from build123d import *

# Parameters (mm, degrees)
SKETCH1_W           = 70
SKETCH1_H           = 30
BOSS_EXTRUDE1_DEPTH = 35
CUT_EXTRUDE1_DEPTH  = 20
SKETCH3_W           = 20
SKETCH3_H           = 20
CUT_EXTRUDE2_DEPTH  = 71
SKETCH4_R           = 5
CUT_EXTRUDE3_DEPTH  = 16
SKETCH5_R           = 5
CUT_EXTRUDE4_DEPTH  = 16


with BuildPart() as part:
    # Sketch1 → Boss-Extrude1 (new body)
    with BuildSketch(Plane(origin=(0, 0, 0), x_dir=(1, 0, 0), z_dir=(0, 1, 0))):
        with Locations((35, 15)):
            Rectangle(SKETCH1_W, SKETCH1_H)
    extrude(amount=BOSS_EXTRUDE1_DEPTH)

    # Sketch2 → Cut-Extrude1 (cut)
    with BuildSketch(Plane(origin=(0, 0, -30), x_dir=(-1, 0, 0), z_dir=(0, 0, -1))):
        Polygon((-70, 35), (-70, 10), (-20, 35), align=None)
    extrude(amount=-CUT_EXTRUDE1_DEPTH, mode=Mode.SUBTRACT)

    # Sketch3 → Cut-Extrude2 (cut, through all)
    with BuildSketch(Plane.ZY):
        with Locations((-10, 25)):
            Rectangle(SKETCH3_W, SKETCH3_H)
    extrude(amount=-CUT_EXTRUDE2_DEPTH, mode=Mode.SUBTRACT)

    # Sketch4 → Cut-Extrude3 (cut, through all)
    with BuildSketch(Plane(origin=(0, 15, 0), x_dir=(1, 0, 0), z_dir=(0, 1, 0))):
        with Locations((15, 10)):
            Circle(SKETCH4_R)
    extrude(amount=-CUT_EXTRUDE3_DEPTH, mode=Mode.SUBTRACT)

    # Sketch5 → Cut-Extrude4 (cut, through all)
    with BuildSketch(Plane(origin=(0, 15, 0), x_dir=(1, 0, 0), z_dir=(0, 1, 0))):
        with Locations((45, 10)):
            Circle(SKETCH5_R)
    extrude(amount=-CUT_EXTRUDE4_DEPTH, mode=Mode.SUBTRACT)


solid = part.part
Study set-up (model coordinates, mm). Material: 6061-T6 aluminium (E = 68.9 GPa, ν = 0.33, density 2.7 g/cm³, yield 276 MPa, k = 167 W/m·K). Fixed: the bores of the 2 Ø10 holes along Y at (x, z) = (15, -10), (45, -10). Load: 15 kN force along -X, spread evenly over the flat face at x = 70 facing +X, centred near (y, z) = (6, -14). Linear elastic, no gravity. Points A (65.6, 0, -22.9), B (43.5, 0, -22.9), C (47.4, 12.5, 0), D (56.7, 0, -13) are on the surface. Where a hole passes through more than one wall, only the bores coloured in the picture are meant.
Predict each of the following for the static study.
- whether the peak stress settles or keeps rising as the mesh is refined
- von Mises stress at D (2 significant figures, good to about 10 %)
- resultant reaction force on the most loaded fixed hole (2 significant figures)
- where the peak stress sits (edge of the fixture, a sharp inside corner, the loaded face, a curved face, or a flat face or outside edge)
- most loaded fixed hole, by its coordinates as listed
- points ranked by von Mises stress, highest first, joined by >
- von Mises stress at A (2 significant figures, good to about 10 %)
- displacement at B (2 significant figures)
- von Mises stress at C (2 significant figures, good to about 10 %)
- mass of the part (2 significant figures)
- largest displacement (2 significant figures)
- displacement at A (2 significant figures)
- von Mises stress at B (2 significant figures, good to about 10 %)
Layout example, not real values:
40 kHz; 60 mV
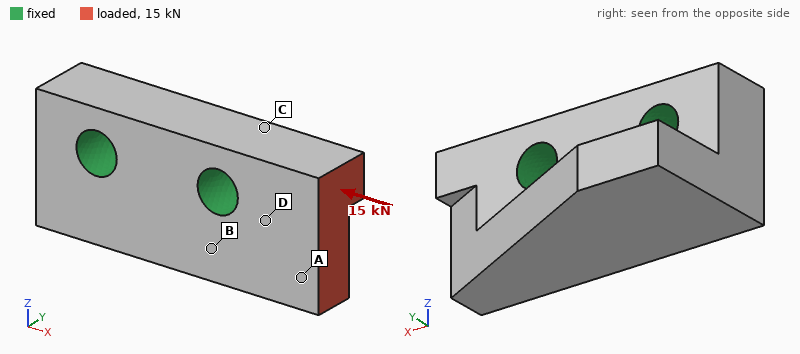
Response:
keeps rising; 62 MPa; 13 kN; edge of the fixture; (45, -10); D > A > B > C; 48 MPa; 5.7 µm; 11 MPa; 99 g; 29 µm; 22 µm; 28 MPa
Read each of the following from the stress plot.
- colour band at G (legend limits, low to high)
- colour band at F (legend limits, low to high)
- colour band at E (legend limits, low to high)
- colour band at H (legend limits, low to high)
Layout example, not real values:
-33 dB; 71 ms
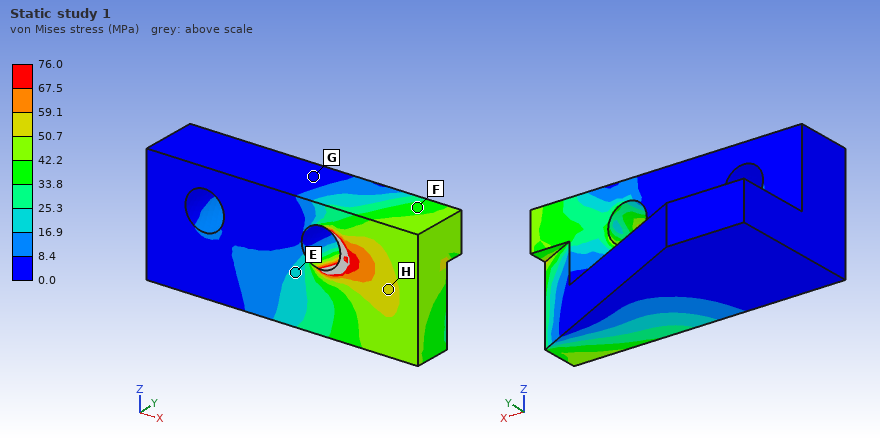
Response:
0.0 to 8.4 MPa; 33.8 to 42.2 MPa; 16.9 to 25.3 MPa; 50.7 to 59.1 MPa
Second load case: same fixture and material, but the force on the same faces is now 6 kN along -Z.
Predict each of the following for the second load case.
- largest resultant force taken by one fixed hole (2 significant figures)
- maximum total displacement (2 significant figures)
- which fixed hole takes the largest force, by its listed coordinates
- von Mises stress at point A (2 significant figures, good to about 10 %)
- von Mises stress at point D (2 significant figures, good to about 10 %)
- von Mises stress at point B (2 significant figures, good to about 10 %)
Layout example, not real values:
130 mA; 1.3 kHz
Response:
8.5 kN; 47 µm; (45, -10); 34 MPa; 39 MPa; 26 MPa
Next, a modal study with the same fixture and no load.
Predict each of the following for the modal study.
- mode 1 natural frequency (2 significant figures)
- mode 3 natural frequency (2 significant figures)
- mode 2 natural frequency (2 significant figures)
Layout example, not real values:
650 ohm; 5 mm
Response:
11 kHz; 19 kHz; 16 kHz
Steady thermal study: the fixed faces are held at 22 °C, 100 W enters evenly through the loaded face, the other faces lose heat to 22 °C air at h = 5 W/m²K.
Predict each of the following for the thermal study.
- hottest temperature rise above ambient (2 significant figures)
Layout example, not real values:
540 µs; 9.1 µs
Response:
35 K
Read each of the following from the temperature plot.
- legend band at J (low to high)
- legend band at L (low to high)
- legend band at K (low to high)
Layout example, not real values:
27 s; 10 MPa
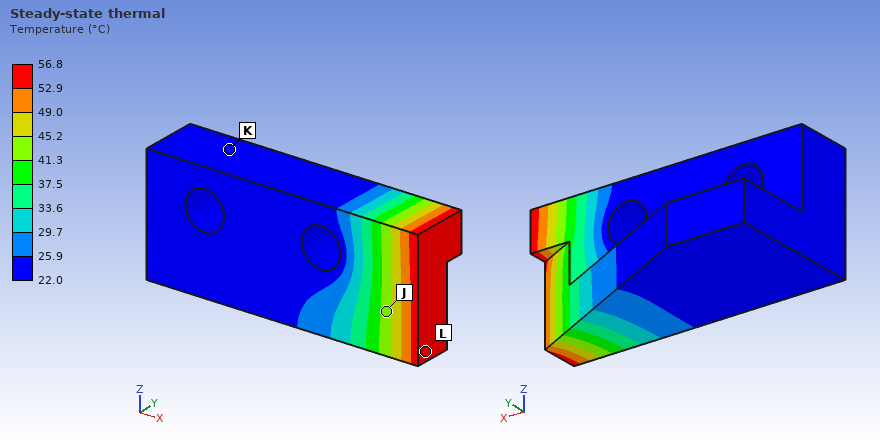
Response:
41.3 to 45.2 °C; 52.9 to 56.8 °C; 22.0 to 25.9 °C
